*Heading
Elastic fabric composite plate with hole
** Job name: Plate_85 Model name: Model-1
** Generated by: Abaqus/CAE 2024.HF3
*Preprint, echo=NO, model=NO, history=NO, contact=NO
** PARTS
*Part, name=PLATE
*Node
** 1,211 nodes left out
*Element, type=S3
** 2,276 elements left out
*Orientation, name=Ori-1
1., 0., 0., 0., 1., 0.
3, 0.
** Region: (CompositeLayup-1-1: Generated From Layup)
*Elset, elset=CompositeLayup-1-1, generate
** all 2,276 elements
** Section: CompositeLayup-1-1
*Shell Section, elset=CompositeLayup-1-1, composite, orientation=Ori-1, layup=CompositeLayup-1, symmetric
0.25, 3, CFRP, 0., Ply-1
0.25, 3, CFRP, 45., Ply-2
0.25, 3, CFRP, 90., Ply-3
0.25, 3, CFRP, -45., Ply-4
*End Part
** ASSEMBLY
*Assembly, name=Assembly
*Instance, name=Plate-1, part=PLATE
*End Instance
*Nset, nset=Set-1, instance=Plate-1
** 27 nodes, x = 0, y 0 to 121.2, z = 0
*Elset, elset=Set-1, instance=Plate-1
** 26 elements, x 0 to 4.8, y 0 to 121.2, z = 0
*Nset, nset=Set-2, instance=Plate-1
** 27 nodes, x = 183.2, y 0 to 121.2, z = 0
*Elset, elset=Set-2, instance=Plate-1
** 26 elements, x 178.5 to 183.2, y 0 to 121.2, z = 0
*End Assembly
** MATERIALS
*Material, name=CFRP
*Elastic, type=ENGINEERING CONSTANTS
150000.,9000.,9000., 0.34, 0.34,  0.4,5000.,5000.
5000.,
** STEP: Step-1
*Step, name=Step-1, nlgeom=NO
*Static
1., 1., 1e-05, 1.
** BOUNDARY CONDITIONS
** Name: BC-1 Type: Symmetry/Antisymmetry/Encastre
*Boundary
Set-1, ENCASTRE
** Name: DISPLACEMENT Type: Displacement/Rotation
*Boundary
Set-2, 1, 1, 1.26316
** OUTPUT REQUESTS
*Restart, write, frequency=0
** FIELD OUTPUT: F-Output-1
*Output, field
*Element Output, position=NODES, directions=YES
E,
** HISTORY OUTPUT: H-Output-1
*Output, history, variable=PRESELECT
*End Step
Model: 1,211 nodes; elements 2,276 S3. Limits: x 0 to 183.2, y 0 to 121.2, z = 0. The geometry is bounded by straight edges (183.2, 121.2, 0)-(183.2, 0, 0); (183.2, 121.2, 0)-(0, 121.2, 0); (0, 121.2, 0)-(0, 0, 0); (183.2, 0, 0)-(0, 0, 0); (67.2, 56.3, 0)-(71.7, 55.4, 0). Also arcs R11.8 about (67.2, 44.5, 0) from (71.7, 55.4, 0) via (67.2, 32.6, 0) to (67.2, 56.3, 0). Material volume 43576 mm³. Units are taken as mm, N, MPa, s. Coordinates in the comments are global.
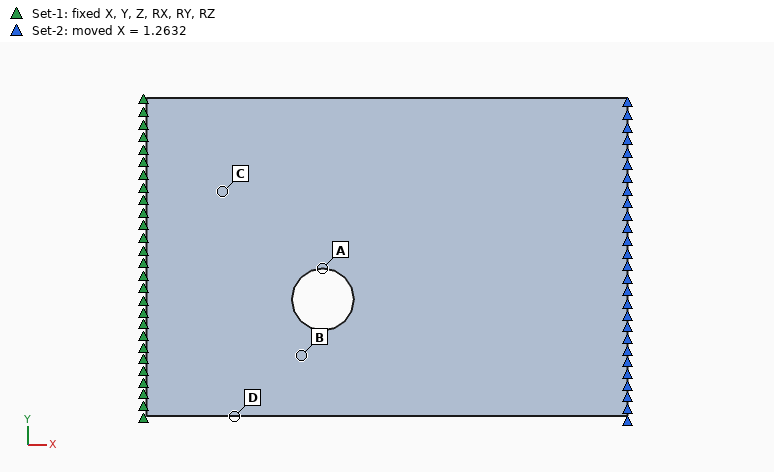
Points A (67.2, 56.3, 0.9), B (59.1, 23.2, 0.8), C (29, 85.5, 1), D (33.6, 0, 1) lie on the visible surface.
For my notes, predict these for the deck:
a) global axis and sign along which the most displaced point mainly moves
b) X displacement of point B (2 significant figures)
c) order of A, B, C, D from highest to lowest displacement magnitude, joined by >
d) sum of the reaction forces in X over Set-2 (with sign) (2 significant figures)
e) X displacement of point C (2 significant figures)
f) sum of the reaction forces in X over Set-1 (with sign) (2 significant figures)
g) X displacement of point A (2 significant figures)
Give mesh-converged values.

+X
0.41 mm
A > B > D > C
91000 N
0.19 mm
-91000 N
0.46 mm
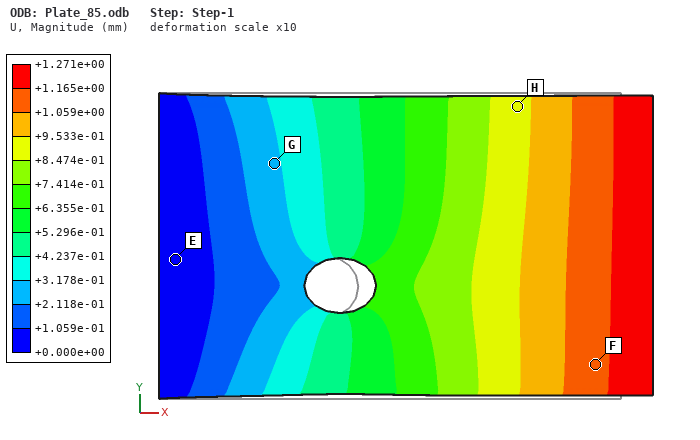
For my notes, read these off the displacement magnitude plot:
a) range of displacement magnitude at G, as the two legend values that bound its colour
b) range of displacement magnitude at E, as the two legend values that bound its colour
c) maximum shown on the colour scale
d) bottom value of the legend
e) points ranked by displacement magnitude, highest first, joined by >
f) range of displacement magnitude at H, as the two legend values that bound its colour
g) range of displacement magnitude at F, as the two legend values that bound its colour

+2.118e-01 to +3.178e-01 mm
+0.000e+00 to +1.059e-01 mm
+1.271e+00 mm
+0.000e+00 mm
F > H > G > E
+8.474e-01 to +9.533e-01 mm
+1.059e+00 to +1.165e+00 mm
